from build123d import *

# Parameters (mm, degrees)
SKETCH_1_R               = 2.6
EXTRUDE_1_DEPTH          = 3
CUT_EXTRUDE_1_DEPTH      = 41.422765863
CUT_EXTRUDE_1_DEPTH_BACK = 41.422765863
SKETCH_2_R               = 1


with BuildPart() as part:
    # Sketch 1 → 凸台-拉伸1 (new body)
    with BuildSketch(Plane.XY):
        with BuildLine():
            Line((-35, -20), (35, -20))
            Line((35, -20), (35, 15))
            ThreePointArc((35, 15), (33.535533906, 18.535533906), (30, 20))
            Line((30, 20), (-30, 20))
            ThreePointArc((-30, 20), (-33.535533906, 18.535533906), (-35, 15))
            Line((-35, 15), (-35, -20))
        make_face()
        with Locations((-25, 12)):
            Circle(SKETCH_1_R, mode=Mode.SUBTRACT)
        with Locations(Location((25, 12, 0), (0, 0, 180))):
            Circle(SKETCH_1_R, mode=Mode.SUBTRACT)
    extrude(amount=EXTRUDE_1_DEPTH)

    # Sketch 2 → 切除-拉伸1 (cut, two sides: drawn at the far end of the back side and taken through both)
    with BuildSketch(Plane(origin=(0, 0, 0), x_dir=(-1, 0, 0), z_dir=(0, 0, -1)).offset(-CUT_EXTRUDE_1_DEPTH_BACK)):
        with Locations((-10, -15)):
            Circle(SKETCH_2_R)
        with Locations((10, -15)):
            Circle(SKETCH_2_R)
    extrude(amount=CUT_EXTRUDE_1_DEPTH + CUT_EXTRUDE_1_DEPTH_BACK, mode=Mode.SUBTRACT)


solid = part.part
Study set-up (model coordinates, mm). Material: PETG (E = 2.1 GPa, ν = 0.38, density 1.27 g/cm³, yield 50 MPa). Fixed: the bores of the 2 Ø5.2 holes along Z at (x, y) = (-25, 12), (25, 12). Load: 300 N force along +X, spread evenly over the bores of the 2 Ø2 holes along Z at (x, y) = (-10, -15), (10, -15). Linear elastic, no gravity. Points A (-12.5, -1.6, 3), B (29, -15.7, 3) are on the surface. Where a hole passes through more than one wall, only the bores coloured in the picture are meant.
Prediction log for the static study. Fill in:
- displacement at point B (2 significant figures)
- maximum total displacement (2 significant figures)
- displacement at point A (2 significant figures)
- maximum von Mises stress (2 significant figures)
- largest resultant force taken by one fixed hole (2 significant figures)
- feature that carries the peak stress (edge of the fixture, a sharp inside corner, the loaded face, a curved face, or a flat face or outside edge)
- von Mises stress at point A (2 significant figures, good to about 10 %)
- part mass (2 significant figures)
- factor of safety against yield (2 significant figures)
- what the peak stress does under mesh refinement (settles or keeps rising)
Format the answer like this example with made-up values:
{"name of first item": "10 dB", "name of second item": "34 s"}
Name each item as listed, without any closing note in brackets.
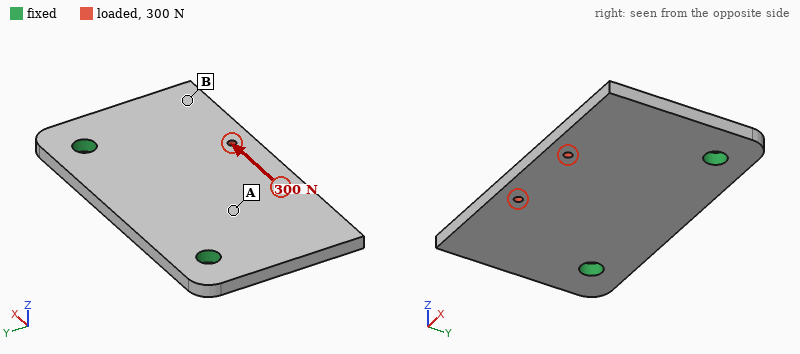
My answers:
{"displacement at point B": "81 µm", "maximum total displacement": "95 µm", "displacement at point A": "42 µm", "maximum von Mises stress": "14 MPa", "largest resultant force taken by one fixed hole": "210 N", "feature that carries the peak stress": "the loaded face", "von Mises stress at point A": "3.3 MPa", "part mass": "10 g", "factor of safety against yield": "3.6", "what the peak stress does under mesh refinement": "settles"}
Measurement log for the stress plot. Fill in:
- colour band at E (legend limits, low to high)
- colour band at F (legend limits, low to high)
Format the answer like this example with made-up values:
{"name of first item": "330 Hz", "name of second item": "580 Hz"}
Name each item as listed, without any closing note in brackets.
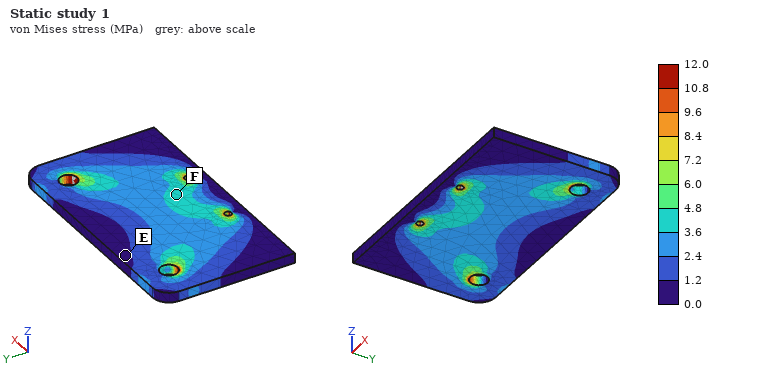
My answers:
{"colour band at E": "0.0 to 1.2 MPa", "colour band at F": "3.6 to 4.8 MPa"}
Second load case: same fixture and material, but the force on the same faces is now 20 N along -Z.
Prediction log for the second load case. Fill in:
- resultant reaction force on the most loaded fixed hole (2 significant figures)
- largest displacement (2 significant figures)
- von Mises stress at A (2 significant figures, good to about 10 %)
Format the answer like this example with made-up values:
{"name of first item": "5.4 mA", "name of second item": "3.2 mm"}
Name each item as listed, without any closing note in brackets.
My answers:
{"resultant reaction force on the most loaded fixed hole": "10 N", "largest displacement": "0.77 mm", "von Mises stress at A": "2.5 MPa"}
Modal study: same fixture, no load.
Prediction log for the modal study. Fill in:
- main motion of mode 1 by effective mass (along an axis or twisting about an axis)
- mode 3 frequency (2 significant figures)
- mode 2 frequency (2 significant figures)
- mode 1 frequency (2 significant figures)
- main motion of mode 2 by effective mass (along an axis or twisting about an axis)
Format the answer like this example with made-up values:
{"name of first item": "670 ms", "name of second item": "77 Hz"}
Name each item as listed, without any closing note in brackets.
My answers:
{"main motion of mode 1 by effective mass": "along Z", "mode 3 frequency": "1400 Hz", "mode 2 frequency": "920 Hz", "mode 1 frequency": "550 Hz", "main motion of mode 2 by effective mass": "twisting about Y"}
